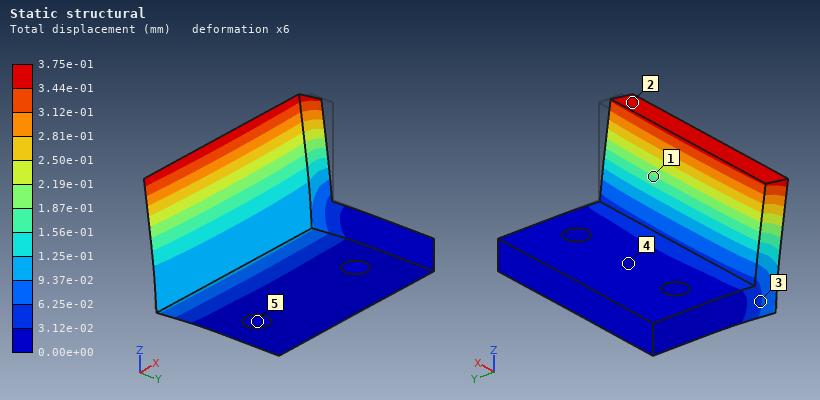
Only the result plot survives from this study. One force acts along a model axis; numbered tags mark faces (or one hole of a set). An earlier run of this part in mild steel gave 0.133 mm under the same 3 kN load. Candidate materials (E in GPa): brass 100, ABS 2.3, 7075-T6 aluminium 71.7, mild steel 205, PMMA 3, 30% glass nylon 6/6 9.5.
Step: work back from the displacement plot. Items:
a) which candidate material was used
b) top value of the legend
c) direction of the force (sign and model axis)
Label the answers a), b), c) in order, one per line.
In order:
a) 7075-T6 aluminium
b) 3.75e-01 mm
c) -Y
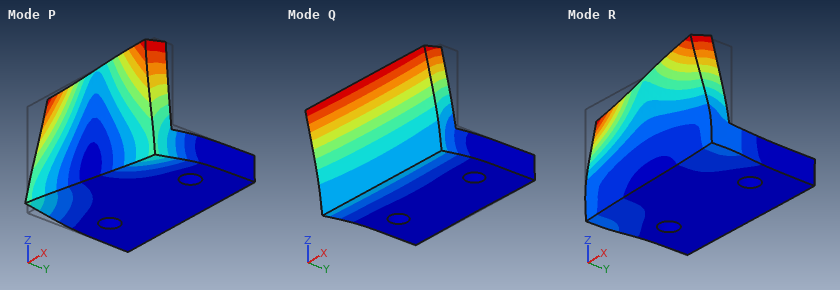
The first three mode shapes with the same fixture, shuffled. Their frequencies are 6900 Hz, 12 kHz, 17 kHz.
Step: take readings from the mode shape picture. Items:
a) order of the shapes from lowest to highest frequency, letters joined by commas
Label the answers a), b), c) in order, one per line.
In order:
a) Q, P, R
